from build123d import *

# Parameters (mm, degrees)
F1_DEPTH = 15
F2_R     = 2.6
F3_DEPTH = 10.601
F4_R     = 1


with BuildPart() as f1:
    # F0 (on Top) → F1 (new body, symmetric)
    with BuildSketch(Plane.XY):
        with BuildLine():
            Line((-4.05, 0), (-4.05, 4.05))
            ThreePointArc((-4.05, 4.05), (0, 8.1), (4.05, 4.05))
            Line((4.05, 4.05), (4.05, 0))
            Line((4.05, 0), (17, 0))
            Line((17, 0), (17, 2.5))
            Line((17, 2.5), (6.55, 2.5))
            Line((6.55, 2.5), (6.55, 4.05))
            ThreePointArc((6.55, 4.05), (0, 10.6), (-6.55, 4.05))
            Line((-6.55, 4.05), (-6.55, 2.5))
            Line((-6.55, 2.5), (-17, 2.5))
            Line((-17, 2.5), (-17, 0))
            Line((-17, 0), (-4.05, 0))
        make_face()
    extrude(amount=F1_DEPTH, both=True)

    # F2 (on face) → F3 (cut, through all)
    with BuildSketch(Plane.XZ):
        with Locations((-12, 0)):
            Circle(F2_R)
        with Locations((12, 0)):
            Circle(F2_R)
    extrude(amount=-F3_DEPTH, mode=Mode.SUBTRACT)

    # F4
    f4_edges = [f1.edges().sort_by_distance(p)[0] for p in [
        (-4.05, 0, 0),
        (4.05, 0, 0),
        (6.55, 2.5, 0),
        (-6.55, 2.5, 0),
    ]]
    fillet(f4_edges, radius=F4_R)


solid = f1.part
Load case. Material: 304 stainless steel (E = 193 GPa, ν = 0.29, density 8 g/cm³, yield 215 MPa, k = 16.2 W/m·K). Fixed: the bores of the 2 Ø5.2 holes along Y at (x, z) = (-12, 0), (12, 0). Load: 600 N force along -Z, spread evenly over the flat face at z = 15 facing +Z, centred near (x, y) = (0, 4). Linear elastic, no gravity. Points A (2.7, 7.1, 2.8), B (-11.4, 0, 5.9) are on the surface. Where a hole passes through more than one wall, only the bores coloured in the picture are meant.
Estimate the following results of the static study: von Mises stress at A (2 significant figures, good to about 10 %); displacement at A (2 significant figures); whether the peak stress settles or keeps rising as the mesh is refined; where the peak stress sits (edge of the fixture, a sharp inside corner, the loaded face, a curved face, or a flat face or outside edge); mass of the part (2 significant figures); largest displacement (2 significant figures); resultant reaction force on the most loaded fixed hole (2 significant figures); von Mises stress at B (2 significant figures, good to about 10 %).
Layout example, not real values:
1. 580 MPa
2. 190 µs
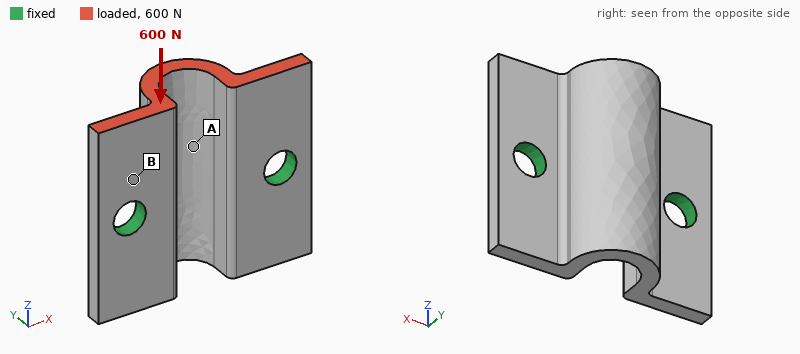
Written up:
1. 3.9 MPa
2. 2.8 µm
3. keeps rising
4. edge of the fixture
5. 27 g
6. 6.6 µm
7. 300 N
8. 13 MPa
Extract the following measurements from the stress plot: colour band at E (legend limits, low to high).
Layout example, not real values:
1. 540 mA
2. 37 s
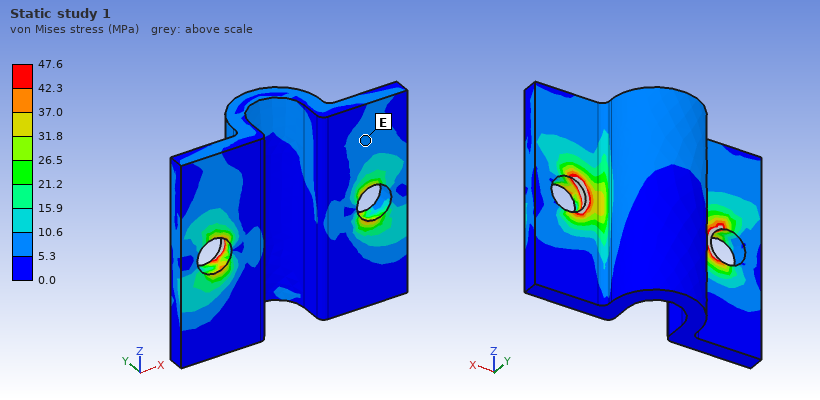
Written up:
1. 5.3 to 10.6 MPa
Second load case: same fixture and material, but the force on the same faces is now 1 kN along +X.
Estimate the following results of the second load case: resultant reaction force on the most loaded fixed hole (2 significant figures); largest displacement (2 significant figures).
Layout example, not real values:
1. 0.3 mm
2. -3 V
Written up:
1. 610 N
2. 11 µm
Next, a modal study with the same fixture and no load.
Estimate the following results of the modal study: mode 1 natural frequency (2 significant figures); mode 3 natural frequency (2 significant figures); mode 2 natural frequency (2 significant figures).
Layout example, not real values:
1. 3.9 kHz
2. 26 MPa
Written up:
1. 7900 Hz
2. 17 kHz
3. 17 kHz
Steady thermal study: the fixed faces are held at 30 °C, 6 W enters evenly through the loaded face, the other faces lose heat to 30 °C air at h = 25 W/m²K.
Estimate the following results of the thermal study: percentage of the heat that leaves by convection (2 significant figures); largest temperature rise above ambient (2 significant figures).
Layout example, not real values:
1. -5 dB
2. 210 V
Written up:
1. 20 %
2. 52 K
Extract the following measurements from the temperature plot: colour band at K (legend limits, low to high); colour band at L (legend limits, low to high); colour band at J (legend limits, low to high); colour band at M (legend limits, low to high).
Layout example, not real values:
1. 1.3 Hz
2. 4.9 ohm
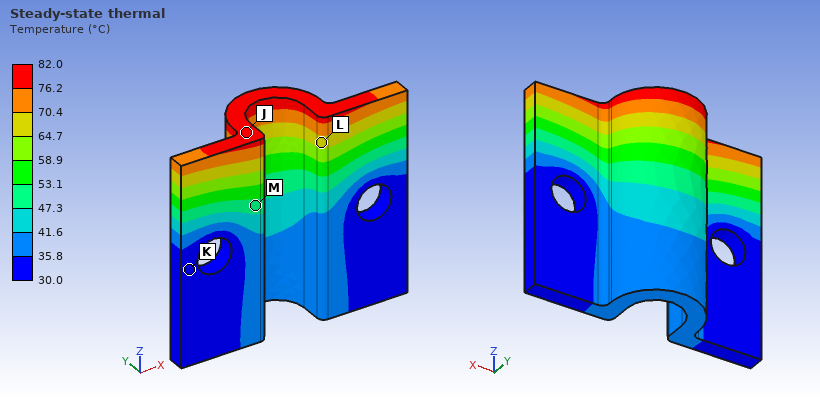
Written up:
1. 30.0 to 35.8 °C
2. 64.7 to 70.4 °C
3. 76.2 to 82.0 °C
4. 47.3 to 53.1 °C
